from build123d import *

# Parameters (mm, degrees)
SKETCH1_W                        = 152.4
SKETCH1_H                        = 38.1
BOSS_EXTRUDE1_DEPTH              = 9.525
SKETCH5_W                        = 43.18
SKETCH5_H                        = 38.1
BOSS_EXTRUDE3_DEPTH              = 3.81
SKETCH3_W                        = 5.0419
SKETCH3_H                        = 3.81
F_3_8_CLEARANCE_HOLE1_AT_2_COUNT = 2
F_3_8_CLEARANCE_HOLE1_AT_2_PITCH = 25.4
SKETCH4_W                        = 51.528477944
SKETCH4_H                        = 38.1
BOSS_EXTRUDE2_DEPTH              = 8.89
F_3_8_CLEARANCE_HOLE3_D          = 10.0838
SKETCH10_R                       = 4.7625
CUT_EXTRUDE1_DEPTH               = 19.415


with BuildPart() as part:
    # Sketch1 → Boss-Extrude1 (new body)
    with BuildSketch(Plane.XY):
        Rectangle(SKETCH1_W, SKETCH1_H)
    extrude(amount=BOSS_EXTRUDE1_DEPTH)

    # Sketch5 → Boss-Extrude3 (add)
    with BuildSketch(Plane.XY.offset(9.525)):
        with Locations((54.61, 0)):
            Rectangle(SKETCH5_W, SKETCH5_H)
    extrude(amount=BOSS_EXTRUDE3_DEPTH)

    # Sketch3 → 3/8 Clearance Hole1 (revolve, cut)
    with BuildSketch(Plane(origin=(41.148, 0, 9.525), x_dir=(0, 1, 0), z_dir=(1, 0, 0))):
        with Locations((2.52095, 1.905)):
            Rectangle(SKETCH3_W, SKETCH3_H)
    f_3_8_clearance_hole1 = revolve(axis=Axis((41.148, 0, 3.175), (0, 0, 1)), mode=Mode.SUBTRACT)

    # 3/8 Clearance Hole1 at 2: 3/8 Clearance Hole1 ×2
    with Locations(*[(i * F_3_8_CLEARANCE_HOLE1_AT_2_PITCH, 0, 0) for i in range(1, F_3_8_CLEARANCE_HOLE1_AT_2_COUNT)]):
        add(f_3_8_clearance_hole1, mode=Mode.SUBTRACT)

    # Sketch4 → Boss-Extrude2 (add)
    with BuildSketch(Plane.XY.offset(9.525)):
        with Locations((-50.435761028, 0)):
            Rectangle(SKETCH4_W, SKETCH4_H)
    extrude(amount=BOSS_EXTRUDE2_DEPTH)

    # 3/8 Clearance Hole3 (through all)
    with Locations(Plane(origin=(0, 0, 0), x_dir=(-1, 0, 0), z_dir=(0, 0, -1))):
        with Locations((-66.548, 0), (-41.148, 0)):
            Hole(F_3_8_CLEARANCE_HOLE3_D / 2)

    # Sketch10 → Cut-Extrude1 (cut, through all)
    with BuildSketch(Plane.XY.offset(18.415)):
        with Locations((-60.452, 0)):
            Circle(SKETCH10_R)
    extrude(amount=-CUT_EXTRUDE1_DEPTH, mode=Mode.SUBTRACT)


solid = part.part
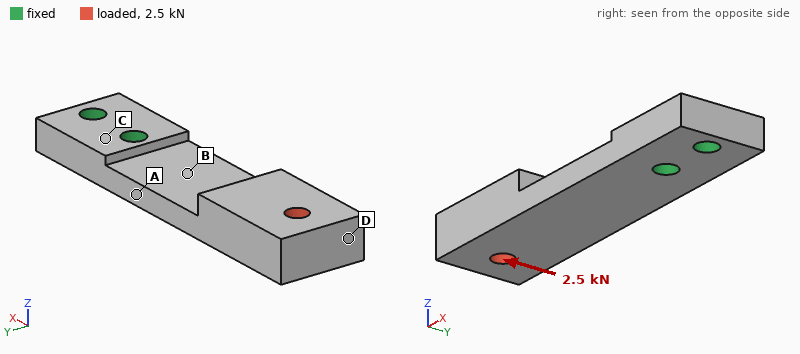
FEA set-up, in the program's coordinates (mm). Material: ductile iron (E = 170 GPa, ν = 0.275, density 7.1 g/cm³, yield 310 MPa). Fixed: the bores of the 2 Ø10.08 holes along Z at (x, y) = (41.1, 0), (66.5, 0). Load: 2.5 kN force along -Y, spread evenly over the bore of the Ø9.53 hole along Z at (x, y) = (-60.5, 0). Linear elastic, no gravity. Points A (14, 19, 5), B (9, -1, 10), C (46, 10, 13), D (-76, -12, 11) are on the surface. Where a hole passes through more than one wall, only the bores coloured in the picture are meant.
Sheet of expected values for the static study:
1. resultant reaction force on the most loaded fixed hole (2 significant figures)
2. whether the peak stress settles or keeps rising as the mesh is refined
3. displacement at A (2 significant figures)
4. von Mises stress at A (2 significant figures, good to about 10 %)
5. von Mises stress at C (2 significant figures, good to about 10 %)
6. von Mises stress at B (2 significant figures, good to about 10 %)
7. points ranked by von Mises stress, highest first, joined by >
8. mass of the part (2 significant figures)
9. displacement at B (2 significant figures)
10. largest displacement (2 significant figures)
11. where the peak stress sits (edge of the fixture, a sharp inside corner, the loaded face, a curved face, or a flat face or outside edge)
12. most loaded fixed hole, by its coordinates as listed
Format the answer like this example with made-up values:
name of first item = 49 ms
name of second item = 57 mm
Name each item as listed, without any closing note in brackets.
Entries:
resultant reaction force on the most loaded fixed hole = 7.8 kN
whether the peak stress settles or keeps rising as the mesh is refined = keeps rising
displacement at A = 0.033 mm
von Mises stress at A = 82 MPa
von Mises stress at C = 25 MPa
von Mises stress at B = 37 MPa
points ranked by von Mises stress, highest first, joined by > = A > B > C > D
mass of the part = 540 g
displacement at B = 0.031 mm
largest displacement = 0.21 mm
where the peak stress sits = edge of the fixture
most loaded fixed hole, by its coordinates as listed = (41.1, 0)
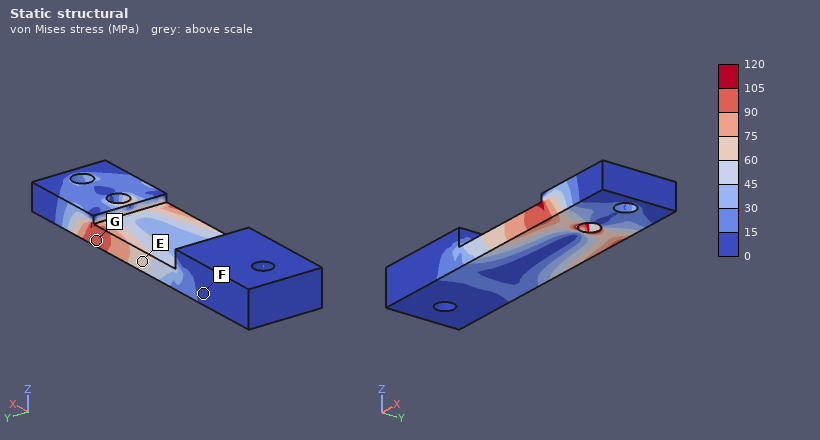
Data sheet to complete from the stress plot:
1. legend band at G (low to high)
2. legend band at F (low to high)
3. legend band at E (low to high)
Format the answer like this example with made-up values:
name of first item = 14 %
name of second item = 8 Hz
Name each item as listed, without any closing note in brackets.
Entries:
legend band at G = 90 to 105 MPa
legend band at F = 0 to 15 MPa
legend band at E = 60 to 75 MPa
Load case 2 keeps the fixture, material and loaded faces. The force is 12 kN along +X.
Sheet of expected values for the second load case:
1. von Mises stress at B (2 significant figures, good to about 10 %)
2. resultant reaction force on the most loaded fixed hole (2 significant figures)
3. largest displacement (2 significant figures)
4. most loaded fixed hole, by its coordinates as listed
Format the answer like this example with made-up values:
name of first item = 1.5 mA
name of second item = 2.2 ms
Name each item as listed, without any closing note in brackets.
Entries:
von Mises stress at B = 120 MPa
resultant reaction force on the most loaded fixed hole = 9.9 kN
largest displacement = 0.60 mm
most loaded fixed hole, by its coordinates as listed = (41.1, 0)
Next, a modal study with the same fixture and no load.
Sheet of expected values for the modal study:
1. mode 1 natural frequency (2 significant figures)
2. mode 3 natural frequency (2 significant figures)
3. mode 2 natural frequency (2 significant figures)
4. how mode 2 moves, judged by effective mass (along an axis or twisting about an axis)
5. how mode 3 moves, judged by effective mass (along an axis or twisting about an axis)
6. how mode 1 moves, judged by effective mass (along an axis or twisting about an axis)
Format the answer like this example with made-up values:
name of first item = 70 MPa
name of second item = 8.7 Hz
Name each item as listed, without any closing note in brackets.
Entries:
mode 1 natural frequency = 440 Hz
mode 3 natural frequency = 2500 Hz
mode 2 natural frequency = 1300 Hz
how mode 2 moves, judged by effective mass = along Y
how mode 3 moves, judged by effective mass = twisting about X
how mode 1 moves, judged by effective mass = along Z
